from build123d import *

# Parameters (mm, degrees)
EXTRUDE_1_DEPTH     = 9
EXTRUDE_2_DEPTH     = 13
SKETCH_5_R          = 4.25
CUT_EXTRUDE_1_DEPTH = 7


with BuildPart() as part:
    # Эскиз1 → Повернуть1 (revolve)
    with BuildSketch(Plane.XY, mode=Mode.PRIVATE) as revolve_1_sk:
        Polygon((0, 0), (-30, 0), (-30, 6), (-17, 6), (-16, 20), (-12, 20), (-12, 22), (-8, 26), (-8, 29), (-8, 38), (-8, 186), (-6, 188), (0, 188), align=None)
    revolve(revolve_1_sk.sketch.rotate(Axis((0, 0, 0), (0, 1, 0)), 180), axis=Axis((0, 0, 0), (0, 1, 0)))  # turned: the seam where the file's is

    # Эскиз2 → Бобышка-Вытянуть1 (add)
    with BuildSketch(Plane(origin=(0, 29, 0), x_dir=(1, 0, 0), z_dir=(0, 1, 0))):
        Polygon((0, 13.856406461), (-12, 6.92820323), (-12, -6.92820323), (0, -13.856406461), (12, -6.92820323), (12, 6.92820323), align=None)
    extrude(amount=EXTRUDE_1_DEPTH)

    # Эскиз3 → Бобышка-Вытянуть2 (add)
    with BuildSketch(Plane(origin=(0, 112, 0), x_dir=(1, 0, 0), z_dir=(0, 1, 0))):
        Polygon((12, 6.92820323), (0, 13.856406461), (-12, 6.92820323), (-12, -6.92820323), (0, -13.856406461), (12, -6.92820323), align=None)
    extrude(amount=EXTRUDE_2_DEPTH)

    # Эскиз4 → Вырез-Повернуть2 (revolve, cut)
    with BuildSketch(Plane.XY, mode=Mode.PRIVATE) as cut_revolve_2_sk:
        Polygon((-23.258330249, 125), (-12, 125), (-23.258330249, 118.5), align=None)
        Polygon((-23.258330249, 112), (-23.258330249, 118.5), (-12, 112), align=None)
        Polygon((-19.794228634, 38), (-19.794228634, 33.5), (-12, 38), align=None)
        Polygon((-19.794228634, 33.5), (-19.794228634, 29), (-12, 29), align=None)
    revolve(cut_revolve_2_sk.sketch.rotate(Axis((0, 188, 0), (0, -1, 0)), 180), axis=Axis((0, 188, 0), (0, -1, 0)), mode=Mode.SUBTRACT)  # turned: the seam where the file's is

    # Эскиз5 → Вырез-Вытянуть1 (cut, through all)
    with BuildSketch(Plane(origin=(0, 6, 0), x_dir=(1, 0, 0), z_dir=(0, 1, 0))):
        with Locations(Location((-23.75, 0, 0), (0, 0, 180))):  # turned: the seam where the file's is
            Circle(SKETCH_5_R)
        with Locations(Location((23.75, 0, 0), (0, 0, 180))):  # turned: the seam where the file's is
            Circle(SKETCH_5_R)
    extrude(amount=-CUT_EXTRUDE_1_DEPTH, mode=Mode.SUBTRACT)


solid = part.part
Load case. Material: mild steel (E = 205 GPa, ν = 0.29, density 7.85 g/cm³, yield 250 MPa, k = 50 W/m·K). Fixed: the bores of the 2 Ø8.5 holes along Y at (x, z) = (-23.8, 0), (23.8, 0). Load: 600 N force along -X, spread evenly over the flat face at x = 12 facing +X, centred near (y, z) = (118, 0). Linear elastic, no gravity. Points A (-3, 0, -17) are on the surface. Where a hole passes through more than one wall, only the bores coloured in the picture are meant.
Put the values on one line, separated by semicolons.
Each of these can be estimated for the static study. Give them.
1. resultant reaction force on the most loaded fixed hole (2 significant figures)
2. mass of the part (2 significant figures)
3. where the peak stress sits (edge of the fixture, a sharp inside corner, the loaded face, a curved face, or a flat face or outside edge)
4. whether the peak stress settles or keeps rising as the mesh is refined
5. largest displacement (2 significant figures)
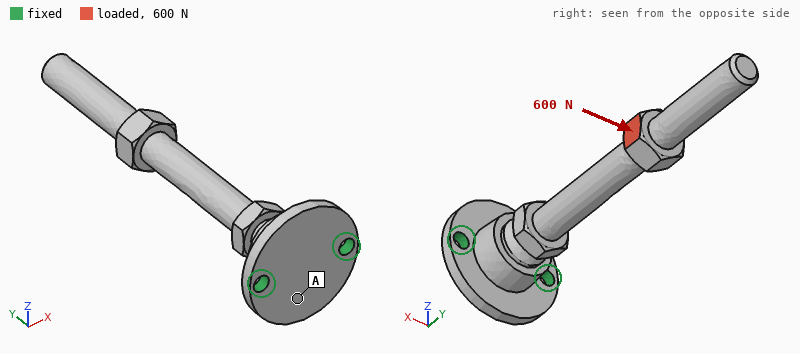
1.9 kN; 540 g; a sharp inside corner; keeps rising; 0.56 mm
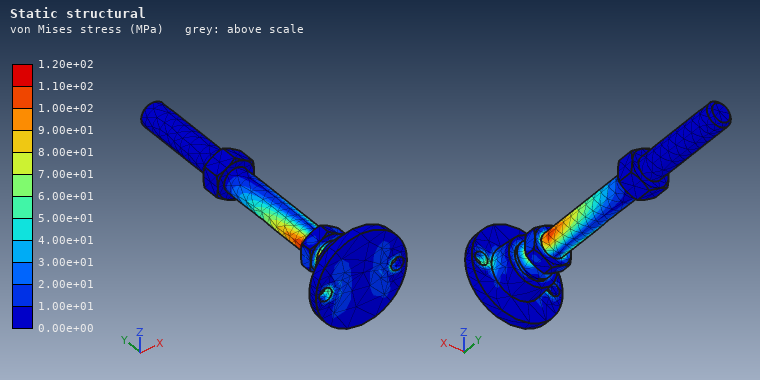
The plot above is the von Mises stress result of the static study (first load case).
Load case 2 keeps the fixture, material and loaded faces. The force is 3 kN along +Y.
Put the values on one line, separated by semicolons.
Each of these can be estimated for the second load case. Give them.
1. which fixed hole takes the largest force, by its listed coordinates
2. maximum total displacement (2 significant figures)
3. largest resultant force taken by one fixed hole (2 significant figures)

(23.8, 0); 0.59 mm; 2.5 kN
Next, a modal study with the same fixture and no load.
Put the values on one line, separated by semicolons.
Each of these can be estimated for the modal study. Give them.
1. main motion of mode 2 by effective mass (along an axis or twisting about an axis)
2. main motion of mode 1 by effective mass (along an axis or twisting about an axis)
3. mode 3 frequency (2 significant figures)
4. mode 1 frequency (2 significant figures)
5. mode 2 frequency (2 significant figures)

along X; along Z; 1900 Hz; 340 Hz; 400 Hz
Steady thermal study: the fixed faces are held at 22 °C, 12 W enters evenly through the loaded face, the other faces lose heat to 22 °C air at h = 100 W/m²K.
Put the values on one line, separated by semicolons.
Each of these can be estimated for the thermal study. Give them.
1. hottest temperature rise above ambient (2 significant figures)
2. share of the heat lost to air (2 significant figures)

31 K; 94 %
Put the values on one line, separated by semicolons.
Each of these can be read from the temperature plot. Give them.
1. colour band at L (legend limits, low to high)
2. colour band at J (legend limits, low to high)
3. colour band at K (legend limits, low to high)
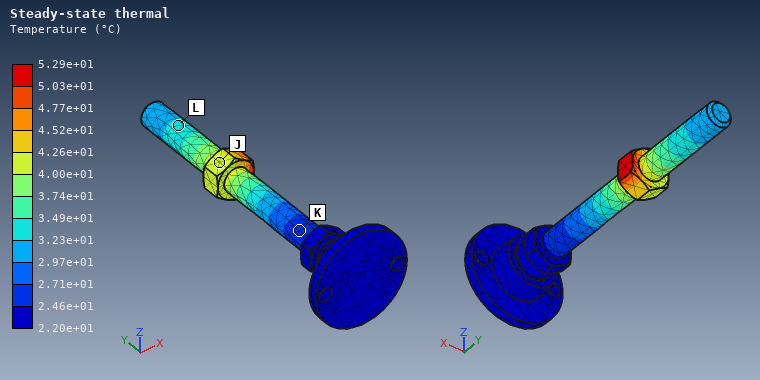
3.23e+01 to 3.49e+01 °C; 4.00e+01 to 4.26e+01 °C; 2.46e+01 to 2.71e+01 °C
